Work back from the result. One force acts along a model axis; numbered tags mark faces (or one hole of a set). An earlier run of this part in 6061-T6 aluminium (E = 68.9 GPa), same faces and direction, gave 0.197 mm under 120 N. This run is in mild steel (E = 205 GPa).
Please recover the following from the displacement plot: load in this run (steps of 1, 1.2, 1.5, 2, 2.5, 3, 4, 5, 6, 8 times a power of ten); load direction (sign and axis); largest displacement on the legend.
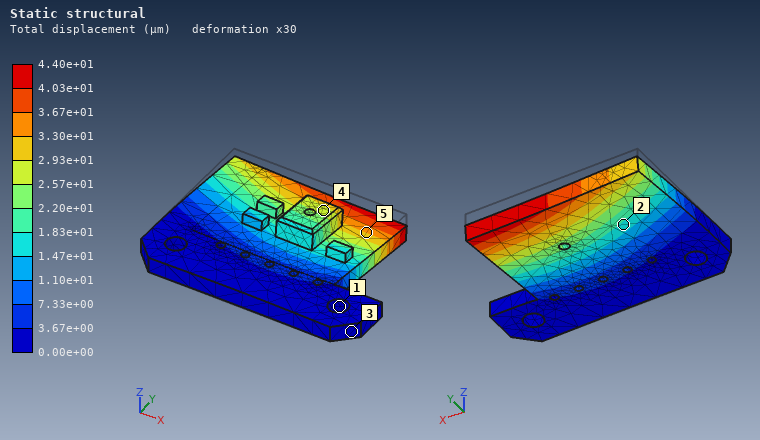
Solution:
80 N
-Z
4.40e+01 µm
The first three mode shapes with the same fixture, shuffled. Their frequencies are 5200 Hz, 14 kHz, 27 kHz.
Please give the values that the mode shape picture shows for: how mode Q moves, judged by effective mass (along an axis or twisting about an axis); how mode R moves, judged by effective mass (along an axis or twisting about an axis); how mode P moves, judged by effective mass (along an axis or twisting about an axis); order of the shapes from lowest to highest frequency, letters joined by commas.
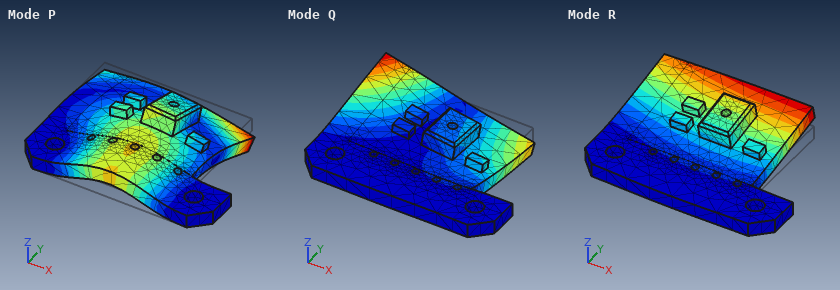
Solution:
twisting about Y
along Z
along Z
R, Q, P
